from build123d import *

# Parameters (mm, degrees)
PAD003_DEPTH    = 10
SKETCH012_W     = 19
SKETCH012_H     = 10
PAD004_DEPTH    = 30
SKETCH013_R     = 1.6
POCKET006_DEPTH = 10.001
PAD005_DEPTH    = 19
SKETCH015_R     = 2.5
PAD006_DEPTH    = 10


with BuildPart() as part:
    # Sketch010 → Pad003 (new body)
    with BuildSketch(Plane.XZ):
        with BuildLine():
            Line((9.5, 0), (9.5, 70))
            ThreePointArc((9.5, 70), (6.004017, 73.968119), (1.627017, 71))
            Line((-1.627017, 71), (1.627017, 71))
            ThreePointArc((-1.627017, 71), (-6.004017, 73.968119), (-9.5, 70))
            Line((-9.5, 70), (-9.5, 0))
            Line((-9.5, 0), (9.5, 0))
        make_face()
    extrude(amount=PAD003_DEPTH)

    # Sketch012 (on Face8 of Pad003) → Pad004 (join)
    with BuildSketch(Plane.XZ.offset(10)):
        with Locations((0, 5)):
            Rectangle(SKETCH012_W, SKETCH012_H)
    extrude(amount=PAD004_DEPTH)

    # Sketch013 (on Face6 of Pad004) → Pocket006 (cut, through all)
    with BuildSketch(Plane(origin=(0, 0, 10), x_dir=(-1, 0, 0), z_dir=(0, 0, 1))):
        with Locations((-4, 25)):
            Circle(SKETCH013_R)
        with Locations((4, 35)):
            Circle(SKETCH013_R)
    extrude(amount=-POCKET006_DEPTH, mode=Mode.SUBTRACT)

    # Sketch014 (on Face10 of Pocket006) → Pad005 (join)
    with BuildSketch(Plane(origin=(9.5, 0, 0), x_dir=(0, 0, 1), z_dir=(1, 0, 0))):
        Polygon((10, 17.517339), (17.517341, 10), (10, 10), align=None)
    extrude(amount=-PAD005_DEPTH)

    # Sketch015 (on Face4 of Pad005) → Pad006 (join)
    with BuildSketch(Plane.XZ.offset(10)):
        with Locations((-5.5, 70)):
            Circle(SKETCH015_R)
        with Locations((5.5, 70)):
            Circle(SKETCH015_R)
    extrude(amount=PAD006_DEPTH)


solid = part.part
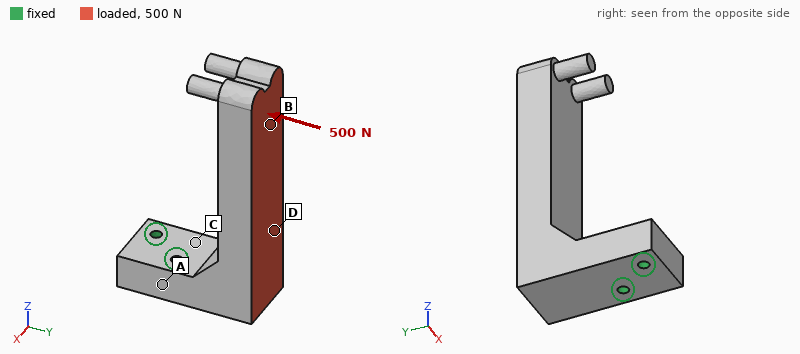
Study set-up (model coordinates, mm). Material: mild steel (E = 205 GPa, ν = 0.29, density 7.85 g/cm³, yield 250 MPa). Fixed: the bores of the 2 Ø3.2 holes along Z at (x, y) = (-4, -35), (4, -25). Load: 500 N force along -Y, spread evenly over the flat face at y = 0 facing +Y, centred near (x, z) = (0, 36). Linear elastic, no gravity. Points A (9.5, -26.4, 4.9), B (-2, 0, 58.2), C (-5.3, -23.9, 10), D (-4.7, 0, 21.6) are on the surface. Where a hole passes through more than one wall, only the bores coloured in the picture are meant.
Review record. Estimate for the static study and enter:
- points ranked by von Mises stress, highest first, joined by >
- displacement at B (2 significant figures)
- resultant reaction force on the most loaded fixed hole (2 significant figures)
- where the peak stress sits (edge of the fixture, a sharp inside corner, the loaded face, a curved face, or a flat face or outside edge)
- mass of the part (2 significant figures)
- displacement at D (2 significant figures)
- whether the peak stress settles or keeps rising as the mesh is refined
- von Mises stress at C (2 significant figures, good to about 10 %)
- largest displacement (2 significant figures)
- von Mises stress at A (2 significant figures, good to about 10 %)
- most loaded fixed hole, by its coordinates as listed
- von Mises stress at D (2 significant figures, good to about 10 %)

C > D > A > B
65 µm
500 N
edge of the fixture
160 g
21 µm
keeps rising
35 MPa
88 µm
14 MPa
(4, -25)
28 MPa
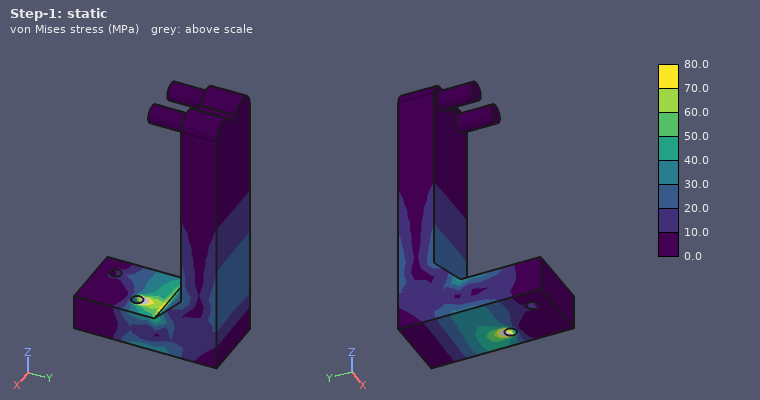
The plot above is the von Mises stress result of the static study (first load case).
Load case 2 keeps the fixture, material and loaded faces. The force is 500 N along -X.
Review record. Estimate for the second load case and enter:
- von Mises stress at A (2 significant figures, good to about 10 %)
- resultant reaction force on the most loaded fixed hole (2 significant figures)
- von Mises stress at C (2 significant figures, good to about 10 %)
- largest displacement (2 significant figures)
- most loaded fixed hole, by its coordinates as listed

18 MPa
1.2 kN
30 MPa
59 µm
(4, -25)
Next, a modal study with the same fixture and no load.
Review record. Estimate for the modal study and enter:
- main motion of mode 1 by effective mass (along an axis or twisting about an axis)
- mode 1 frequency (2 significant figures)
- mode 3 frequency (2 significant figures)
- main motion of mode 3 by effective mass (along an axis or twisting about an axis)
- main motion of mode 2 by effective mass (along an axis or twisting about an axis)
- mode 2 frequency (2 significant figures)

along Y
1300 Hz
5300 Hz
along Z
along X
1700 Hz
